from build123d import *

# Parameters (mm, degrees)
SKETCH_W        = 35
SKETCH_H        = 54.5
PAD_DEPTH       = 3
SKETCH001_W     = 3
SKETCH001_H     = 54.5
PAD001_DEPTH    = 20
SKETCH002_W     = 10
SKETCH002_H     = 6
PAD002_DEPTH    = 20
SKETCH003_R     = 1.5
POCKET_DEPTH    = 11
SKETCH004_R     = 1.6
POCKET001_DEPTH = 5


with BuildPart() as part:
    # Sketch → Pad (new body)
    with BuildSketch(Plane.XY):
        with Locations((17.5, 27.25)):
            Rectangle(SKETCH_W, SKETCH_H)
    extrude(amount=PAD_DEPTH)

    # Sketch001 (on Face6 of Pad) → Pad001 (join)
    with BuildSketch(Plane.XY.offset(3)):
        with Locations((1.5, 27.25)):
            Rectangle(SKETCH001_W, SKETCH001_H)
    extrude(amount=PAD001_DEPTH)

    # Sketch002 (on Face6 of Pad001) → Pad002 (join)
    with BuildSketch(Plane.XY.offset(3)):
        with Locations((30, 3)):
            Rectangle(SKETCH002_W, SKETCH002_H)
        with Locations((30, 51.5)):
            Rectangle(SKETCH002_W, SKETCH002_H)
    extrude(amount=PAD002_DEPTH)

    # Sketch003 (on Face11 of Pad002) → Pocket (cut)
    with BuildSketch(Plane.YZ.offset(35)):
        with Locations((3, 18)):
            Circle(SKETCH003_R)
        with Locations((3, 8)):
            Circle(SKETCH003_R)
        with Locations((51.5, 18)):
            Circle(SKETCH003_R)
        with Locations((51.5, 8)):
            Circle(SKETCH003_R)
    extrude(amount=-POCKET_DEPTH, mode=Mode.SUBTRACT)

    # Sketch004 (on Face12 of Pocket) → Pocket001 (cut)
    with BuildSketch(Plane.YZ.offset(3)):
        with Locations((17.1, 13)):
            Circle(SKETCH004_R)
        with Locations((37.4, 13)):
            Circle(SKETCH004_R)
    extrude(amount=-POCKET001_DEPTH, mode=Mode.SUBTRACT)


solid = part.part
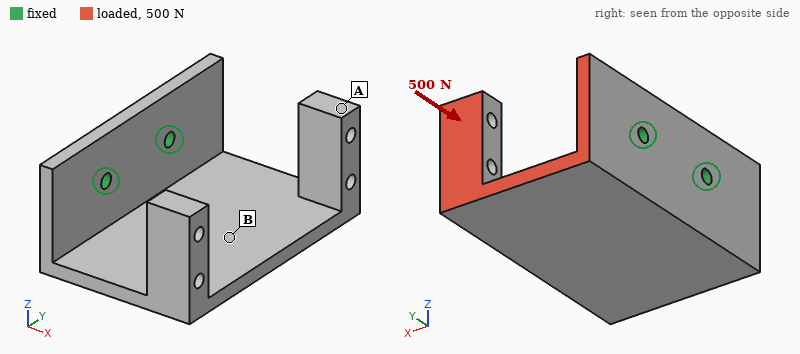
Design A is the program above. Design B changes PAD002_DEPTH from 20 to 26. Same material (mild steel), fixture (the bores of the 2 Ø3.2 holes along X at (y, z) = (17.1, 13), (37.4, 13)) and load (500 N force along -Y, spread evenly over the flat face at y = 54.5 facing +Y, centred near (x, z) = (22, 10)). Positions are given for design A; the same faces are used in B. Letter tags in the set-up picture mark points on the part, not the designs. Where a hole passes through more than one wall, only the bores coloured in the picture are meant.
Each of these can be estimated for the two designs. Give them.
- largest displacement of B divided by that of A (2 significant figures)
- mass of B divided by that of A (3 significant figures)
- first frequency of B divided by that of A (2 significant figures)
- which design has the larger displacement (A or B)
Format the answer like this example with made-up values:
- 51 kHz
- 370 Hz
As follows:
- 1.6
- 1.07
- 0.88
- B
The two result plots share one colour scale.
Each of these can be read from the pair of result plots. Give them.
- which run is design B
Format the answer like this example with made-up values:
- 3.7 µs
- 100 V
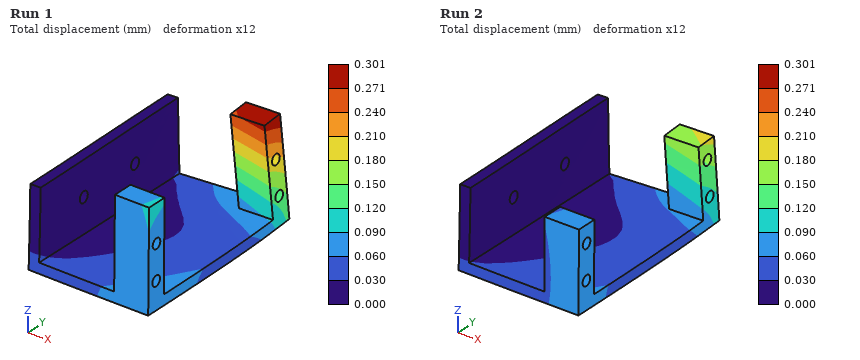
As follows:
- Run 1
